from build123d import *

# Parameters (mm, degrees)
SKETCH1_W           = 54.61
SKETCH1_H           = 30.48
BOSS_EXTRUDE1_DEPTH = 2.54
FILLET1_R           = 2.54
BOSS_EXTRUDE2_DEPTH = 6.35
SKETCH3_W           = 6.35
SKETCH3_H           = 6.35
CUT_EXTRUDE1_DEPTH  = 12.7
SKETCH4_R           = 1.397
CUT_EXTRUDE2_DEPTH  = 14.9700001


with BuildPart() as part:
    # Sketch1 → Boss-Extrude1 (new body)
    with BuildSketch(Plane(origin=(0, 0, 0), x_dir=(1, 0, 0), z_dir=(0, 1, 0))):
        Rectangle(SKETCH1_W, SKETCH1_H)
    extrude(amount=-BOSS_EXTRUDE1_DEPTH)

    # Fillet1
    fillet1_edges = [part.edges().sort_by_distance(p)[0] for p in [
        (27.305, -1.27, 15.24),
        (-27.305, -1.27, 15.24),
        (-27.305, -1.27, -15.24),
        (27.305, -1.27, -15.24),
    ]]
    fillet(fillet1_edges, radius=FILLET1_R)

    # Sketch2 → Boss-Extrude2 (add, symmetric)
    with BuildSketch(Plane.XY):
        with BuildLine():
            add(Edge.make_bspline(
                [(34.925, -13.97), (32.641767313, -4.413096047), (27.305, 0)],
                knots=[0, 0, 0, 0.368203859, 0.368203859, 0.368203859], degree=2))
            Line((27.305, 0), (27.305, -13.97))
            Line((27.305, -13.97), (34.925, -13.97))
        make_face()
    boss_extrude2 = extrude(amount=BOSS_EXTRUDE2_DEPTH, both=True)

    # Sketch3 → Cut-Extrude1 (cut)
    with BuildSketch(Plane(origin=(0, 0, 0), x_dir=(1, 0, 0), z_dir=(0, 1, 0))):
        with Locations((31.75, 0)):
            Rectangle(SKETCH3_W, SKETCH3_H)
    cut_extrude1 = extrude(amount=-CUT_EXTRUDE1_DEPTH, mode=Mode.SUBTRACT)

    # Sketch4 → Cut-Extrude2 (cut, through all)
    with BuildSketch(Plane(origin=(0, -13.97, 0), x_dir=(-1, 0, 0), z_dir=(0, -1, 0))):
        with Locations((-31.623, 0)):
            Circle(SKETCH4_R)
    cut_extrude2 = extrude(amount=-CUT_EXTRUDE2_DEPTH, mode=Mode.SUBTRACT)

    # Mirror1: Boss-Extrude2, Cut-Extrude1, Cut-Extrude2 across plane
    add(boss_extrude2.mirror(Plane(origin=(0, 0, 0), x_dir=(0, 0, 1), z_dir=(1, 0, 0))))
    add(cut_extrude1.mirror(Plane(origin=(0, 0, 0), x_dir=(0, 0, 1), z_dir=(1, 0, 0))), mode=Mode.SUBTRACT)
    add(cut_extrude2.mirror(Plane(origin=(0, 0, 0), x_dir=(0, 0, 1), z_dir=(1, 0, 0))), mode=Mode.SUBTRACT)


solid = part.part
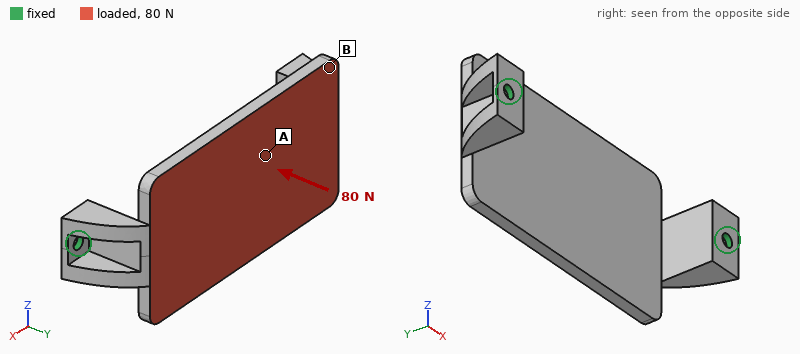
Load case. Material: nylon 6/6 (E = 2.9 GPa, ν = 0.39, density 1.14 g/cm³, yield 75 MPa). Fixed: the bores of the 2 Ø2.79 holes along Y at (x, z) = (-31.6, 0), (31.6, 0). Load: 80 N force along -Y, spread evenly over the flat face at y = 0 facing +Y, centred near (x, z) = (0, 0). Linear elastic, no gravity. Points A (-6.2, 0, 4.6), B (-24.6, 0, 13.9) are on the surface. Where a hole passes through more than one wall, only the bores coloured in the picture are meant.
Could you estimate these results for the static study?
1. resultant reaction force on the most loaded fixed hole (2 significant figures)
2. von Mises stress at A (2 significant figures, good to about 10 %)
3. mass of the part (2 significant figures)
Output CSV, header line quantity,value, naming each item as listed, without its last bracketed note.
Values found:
quantity,value
resultant reaction force on the most loaded fixed hole,52 N
von Mises stress at A,9.1 MPa
mass of the part,6.1 g
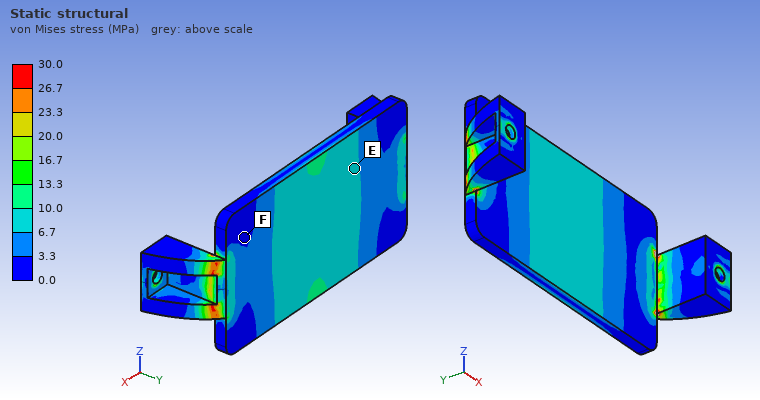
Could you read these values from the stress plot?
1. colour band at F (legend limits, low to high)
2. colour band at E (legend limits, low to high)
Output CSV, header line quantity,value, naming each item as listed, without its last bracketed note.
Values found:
quantity,value
colour band at F,0.0 to 3.3 MPa
colour band at E,6.7 to 10.0 MPa
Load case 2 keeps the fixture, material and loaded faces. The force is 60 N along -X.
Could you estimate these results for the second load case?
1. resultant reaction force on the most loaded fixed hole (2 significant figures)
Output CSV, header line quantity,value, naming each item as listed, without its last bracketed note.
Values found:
quantity,value
resultant reaction force on the most loaded fixed hole,31 N
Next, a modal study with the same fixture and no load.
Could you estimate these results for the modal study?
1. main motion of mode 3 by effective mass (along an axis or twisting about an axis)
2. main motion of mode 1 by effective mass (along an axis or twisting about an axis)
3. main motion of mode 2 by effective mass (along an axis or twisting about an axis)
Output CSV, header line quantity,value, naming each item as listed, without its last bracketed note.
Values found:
quantity,value
main motion of mode 3 by effective mass,along X
main motion of mode 1 by effective mass,along Z
main motion of mode 2 by effective mass,along Y
